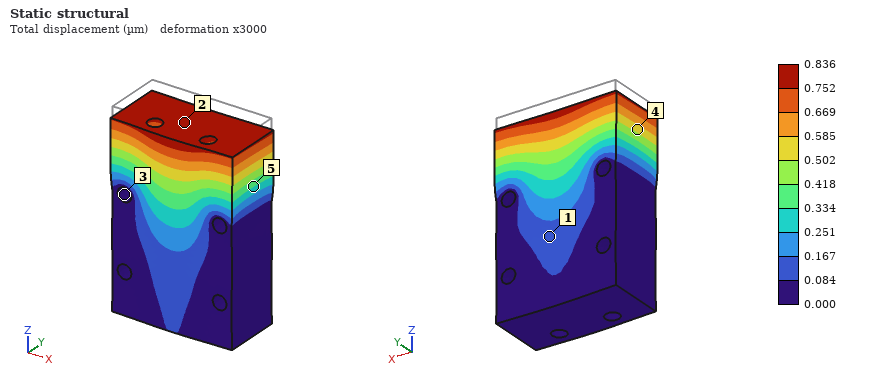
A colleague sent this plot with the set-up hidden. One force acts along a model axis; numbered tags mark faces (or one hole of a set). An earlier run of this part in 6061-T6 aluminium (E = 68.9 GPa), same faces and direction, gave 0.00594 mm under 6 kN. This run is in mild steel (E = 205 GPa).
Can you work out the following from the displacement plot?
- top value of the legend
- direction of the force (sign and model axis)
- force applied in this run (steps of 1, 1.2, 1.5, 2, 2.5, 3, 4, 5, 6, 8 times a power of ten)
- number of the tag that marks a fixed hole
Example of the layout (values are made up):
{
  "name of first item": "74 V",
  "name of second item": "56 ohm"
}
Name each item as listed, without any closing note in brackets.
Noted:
{
  "top value of the legend": "0.836 µm",
  "direction of the force": "-Z",
  "force applied in this run": "2.5 kN",
  "number of the tag that marks a fixed hole": "3"
}
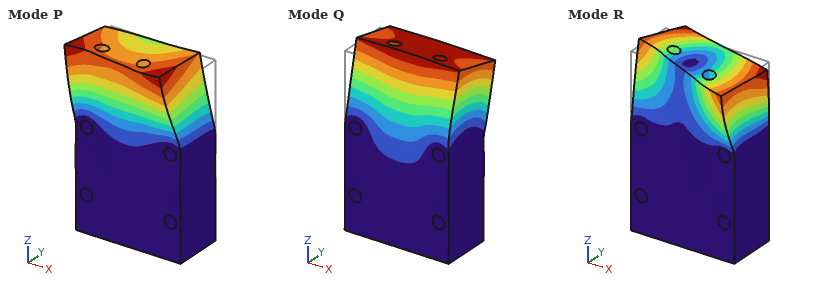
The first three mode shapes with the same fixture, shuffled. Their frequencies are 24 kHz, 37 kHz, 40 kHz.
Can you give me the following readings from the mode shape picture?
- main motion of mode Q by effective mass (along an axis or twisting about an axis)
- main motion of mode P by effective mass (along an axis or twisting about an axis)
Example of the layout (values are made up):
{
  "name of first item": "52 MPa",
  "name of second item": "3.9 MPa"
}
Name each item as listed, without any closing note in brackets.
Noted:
{
  "main motion of mode Q by effective mass": "along Y",
  "main motion of mode P by effective mass": "along X"
}
